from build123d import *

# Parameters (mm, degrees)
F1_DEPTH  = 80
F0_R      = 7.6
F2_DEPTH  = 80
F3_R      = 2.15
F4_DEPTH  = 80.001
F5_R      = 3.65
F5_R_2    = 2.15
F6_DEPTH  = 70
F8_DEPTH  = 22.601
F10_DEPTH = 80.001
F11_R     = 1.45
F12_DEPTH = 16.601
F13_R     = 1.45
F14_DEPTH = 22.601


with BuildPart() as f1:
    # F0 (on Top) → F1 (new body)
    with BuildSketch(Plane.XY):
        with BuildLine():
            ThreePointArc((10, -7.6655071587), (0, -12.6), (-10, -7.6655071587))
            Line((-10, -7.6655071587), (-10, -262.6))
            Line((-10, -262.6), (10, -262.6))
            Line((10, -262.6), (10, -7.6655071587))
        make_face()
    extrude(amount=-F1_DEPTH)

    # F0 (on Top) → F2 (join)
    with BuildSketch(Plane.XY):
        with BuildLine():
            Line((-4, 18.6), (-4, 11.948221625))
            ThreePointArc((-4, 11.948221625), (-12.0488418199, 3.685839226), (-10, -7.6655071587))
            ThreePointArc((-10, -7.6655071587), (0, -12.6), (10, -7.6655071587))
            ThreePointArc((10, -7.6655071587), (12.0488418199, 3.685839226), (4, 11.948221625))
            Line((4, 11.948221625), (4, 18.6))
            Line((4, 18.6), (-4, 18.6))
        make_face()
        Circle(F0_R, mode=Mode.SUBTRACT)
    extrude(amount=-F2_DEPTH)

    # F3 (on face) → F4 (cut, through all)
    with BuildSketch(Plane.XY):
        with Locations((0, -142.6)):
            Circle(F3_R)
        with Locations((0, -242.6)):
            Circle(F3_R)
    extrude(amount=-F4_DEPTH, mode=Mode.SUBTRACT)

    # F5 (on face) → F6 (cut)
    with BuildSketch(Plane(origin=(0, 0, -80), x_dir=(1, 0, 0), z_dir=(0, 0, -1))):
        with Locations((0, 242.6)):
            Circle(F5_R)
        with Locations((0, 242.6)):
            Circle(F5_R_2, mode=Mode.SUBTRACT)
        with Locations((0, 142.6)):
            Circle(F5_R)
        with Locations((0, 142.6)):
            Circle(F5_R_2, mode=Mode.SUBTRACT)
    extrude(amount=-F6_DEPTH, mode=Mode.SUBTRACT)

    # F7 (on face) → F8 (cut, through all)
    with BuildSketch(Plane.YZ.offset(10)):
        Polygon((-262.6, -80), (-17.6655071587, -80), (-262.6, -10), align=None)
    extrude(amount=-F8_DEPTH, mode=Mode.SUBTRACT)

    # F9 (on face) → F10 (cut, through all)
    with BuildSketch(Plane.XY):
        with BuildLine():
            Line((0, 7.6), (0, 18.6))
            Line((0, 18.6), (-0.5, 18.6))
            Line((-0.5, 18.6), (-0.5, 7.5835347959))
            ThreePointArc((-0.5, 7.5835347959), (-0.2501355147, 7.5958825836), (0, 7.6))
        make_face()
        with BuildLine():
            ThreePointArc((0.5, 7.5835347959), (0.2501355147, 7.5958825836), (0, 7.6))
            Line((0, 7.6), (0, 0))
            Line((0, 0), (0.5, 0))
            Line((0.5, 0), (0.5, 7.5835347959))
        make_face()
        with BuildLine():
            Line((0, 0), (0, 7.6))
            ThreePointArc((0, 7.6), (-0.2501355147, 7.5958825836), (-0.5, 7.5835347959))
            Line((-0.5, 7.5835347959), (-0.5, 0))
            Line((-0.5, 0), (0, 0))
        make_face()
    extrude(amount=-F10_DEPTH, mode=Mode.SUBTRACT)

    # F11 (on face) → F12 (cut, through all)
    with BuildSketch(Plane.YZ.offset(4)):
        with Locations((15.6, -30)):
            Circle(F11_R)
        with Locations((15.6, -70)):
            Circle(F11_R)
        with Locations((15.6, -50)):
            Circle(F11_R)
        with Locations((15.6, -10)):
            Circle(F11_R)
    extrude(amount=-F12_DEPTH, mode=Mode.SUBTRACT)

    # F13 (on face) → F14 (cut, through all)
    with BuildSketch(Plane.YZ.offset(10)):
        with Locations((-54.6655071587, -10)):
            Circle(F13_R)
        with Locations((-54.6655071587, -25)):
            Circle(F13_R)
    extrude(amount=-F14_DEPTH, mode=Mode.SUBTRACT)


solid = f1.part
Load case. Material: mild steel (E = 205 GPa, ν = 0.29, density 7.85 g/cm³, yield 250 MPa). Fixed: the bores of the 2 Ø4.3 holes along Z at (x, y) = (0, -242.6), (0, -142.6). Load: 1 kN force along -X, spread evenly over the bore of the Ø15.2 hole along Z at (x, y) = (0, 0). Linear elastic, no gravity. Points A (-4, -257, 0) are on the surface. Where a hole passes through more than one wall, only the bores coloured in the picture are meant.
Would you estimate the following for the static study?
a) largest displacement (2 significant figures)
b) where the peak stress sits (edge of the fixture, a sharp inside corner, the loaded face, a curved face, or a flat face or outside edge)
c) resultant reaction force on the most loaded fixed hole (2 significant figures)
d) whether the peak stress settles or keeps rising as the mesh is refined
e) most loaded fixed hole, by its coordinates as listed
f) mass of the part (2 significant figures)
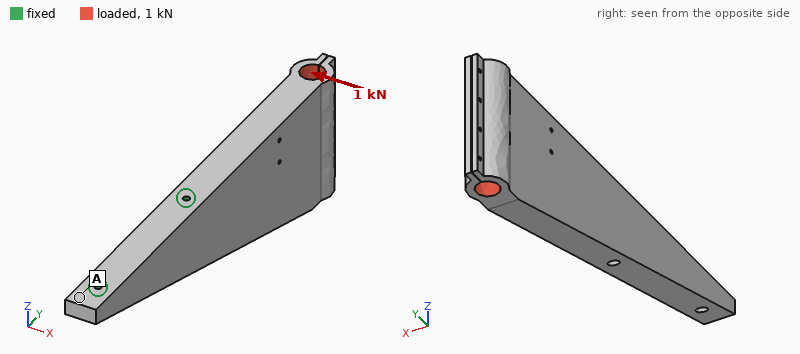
0.33 mm
edge of the fixture
2.2 kN
keeps rising
(0, -142.6)
2.0 kg
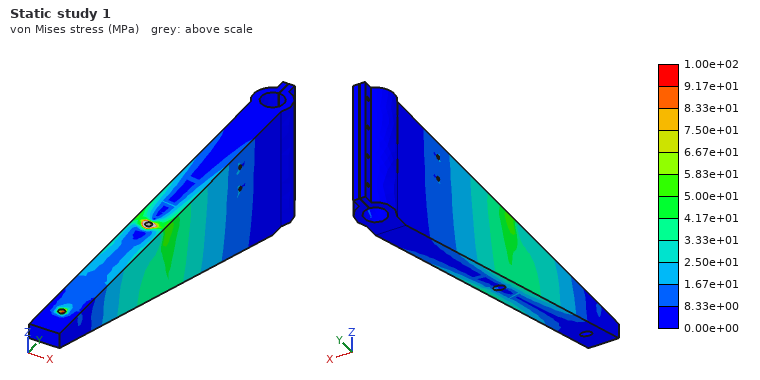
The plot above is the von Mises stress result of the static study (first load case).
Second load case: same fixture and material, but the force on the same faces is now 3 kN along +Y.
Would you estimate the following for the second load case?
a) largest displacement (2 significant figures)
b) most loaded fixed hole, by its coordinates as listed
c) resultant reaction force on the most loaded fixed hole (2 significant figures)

39 µm
(0, -242.6)
2.4 kN
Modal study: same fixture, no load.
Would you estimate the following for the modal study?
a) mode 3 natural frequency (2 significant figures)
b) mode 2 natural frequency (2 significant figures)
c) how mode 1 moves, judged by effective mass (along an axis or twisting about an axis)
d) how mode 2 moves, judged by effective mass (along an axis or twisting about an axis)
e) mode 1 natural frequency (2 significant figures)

1400 Hz
820 Hz
along X
along Z
400 Hz
